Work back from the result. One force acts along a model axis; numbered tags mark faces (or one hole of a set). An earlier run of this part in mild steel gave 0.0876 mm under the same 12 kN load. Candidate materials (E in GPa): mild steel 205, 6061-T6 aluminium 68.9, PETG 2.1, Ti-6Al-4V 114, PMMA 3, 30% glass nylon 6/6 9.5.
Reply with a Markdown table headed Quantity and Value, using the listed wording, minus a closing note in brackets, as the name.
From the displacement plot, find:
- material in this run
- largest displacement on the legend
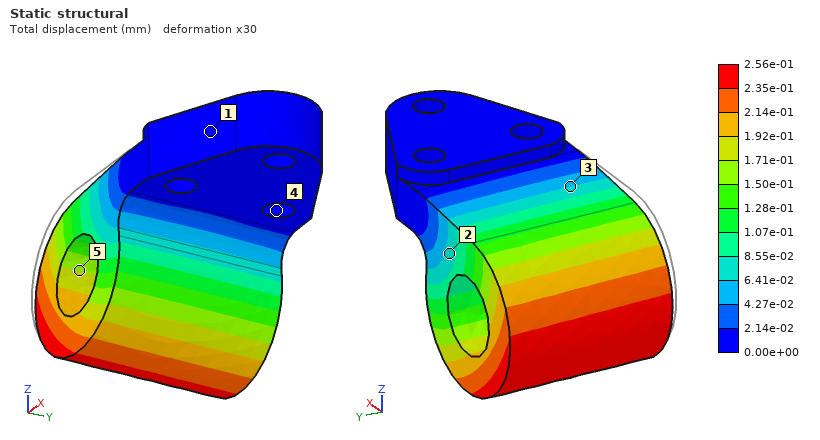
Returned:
| Quantity | Value |
|---|---|
| material in this run | 6061-T6 aluminium |
| largest displacement on the legend | 2.56e-01 mm |
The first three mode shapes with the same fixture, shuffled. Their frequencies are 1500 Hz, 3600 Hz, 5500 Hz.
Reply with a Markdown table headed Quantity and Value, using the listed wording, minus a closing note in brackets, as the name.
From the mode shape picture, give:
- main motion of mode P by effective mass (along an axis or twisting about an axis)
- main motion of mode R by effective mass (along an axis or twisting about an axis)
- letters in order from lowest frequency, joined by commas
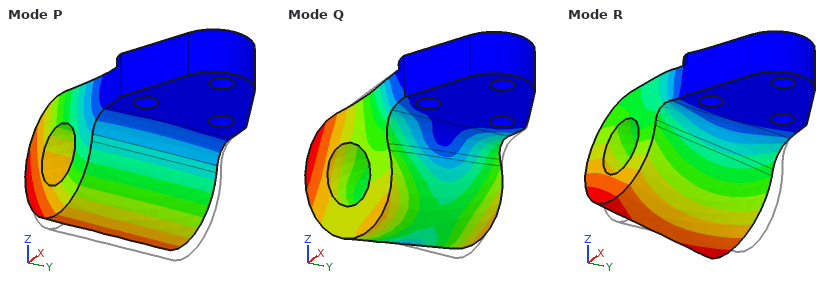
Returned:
| Quantity | Value |
|---|---|
| main motion of mode P by effective mass | along Z |
| main motion of mode R by effective mass | along Y |
| letters in order from lowest frequency, joined by commas | P, R, Q |
